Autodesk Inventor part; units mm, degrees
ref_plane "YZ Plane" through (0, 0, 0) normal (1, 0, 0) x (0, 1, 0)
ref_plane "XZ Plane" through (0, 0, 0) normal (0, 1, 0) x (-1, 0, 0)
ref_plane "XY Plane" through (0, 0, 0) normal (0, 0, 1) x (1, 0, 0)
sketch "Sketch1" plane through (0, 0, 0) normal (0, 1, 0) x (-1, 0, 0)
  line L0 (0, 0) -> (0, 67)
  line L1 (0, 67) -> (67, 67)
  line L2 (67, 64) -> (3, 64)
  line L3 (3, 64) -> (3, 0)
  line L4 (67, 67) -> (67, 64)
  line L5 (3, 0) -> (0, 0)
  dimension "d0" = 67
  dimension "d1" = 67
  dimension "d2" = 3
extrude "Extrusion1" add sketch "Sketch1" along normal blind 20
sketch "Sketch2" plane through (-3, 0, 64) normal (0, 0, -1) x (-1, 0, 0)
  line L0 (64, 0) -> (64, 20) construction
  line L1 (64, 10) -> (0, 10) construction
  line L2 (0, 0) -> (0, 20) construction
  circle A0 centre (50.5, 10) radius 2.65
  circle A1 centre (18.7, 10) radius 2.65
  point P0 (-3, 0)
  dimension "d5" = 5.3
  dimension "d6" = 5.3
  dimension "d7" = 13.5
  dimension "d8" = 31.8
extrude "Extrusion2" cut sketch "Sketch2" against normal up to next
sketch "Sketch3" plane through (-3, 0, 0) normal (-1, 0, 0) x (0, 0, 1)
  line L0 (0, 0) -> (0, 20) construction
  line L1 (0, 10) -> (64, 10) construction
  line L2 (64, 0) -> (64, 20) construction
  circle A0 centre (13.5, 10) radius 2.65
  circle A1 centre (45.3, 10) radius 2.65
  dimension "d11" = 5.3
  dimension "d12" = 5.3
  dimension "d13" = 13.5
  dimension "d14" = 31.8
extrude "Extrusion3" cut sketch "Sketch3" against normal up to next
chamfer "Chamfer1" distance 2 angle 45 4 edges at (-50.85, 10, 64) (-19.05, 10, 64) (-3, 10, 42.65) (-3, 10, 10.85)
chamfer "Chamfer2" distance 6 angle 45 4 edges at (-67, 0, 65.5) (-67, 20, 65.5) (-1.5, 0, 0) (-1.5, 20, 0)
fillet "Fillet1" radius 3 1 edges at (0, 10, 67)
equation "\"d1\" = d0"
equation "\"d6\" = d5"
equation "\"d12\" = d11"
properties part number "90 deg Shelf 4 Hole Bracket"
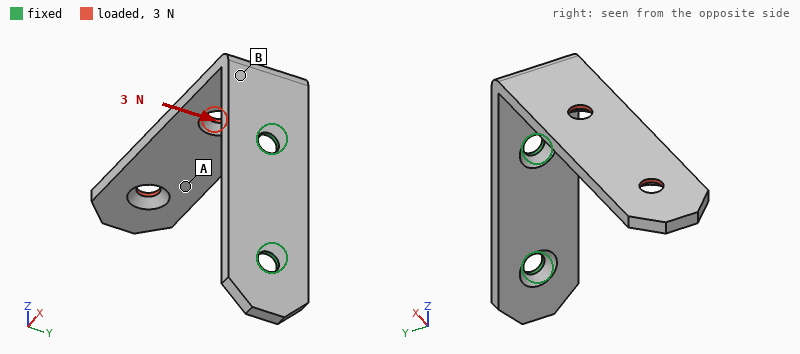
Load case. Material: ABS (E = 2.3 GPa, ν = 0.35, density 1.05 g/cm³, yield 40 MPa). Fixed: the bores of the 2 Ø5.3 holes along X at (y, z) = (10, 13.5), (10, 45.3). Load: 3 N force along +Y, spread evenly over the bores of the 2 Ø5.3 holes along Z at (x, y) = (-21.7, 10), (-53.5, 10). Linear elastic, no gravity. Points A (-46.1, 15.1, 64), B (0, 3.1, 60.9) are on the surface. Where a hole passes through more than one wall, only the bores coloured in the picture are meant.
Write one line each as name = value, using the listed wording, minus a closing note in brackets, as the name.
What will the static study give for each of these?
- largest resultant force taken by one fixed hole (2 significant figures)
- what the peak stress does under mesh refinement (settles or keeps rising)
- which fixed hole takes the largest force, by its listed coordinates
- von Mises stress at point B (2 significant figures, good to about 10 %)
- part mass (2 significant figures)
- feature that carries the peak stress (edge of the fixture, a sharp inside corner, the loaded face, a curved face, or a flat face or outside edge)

largest resultant force taken by one fixed hole = 3.5 N
what the peak stress does under mesh refinement = keeps rising
which fixed hole takes the largest force, by its listed coordinates = (10, 45.3)
von Mises stress at point B = 2.5 MPa
part mass = 7.5 g
feature that carries the peak stress = edge of the fixture
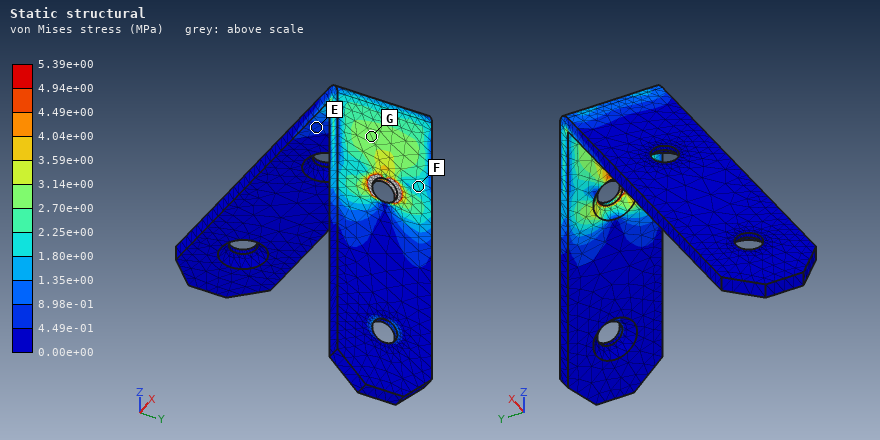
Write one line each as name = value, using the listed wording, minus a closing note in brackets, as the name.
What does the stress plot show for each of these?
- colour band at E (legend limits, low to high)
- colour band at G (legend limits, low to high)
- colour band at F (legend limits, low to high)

colour band at E = 4.49e-01 to 8.98e-01 MPa
colour band at G = 2.70e+00 to 3.14e+00 MPa
colour band at F = 1.80e+00 to 2.25e+00 MPa
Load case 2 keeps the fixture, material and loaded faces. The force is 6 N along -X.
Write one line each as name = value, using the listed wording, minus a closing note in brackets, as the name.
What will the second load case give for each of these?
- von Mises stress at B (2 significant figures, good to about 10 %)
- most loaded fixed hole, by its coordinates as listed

von Mises stress at B = 1.1 MPa
most loaded fixed hole, by its coordinates as listed = (10, 45.3)
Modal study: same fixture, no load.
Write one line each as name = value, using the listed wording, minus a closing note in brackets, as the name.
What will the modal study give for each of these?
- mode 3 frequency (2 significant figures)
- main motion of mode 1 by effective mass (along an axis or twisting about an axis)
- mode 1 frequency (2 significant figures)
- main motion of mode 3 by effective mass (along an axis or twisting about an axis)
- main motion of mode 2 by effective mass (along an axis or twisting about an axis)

mode 3 frequency = 520 Hz
main motion of mode 1 by effective mass = along Z
mode 1 frequency = 110 Hz
main motion of mode 3 by effective mass = along X
main motion of mode 2 by effective mass = along Y
